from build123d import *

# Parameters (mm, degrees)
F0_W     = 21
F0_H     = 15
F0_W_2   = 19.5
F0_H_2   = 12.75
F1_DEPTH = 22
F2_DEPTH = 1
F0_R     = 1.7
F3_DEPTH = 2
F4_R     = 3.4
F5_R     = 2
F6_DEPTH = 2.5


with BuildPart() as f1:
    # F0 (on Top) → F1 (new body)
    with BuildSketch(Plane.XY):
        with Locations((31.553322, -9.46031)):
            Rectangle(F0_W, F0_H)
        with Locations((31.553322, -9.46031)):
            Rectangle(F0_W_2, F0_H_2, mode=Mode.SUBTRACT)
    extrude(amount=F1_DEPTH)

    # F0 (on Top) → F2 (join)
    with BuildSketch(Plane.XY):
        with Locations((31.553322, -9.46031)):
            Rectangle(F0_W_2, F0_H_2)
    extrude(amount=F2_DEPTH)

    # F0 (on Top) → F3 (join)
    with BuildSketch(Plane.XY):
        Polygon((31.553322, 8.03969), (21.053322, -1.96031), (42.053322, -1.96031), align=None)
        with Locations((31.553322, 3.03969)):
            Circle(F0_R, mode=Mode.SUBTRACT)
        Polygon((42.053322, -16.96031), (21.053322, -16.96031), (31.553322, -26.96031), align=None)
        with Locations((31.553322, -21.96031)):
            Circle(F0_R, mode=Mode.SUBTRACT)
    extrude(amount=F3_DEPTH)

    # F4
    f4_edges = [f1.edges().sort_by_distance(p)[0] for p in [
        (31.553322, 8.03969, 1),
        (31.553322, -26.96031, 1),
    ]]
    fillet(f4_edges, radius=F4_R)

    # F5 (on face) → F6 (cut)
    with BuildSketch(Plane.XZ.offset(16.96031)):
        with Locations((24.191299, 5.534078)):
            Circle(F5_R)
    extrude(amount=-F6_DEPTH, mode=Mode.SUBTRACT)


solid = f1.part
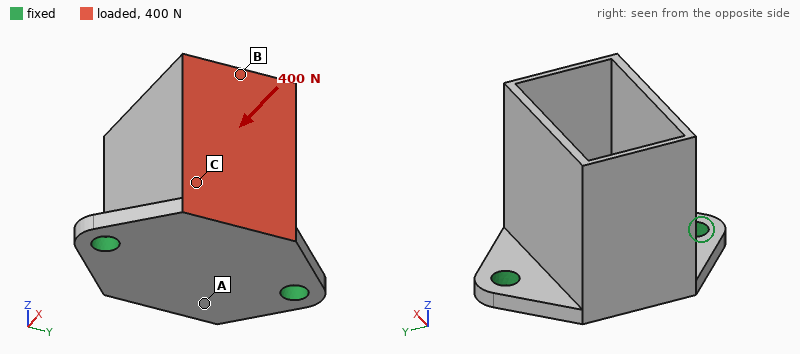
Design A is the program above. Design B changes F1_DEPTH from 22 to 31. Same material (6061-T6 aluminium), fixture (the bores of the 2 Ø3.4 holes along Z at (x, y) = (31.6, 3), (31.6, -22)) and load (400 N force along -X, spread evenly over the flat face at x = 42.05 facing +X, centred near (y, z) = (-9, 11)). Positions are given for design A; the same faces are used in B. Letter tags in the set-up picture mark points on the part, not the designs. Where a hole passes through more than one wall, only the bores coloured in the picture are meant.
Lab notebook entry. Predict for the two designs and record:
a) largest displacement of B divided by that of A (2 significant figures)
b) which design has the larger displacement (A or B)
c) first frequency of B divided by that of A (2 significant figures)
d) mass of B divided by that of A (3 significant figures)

1.6
B
0.64
1.29
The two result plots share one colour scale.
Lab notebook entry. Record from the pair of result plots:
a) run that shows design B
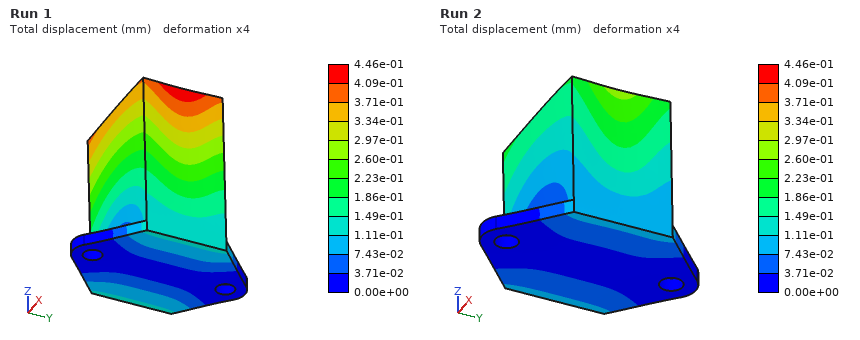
Run 1
